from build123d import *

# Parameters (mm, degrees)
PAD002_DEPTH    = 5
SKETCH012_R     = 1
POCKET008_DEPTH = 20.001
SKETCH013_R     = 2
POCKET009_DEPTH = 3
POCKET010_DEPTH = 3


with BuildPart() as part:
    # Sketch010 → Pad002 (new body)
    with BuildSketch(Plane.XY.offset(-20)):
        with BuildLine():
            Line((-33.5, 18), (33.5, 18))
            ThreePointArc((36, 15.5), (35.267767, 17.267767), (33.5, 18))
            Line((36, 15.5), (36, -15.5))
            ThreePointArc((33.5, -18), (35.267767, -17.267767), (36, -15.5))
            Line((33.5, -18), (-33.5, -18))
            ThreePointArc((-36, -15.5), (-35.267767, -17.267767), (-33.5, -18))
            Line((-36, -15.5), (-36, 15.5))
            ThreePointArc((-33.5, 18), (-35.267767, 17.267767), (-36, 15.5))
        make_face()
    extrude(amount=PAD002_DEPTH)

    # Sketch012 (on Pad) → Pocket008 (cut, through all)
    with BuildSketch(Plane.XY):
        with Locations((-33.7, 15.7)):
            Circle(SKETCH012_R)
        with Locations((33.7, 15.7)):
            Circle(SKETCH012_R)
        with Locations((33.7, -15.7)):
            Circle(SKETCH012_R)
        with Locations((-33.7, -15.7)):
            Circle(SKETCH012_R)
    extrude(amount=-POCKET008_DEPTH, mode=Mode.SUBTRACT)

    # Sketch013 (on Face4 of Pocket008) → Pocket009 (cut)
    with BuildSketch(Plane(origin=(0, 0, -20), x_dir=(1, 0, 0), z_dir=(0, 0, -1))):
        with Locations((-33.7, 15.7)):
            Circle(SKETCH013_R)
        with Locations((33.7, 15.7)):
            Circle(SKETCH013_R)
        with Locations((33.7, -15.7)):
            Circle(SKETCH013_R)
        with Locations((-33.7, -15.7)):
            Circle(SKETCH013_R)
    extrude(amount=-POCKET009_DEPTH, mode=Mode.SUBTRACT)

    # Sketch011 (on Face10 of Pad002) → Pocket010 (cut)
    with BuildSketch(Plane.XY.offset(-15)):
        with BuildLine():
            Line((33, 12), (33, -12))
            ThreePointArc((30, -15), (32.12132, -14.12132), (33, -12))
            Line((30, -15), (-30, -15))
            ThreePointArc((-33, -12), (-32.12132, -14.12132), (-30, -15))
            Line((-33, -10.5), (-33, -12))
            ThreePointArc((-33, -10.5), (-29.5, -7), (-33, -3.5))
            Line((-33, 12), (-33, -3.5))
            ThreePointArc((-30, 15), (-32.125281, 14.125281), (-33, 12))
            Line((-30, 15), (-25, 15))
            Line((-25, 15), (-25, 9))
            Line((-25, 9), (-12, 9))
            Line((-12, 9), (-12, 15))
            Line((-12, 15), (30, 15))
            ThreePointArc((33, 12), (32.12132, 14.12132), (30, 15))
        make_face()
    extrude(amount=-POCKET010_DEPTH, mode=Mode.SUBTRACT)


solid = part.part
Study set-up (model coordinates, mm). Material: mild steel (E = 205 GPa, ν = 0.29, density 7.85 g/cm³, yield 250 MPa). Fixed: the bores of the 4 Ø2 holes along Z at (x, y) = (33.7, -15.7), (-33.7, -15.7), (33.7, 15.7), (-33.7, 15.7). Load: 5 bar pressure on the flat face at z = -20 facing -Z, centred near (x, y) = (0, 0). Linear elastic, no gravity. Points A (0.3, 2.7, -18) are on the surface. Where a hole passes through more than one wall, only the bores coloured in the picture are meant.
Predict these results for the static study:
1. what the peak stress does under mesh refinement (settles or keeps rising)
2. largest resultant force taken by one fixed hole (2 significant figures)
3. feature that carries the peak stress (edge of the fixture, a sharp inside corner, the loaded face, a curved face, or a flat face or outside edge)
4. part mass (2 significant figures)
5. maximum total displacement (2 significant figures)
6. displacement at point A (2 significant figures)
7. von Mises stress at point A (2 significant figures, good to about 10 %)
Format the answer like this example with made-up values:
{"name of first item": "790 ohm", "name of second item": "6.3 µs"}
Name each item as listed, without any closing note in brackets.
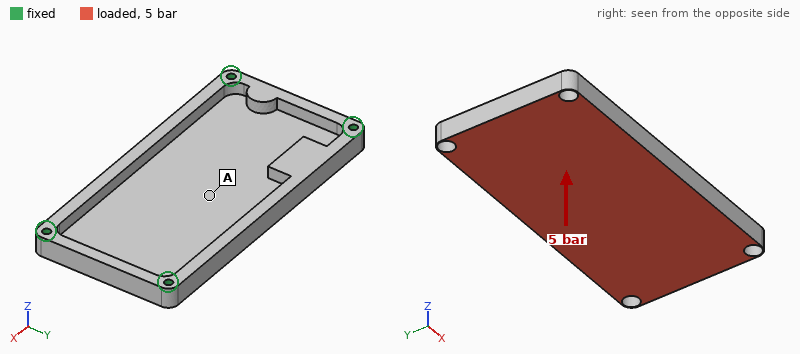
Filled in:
{"what the peak stress does under mesh refinement": "keeps rising", "largest resultant force taken by one fixed hole": "790 N", "feature that carries the peak stress": "edge of the fixture", "part mass": "56 g", "maximum total displacement": "78 µm", "displacement at point A": "77 µm", "von Mises stress at point A": "41 MPa"}
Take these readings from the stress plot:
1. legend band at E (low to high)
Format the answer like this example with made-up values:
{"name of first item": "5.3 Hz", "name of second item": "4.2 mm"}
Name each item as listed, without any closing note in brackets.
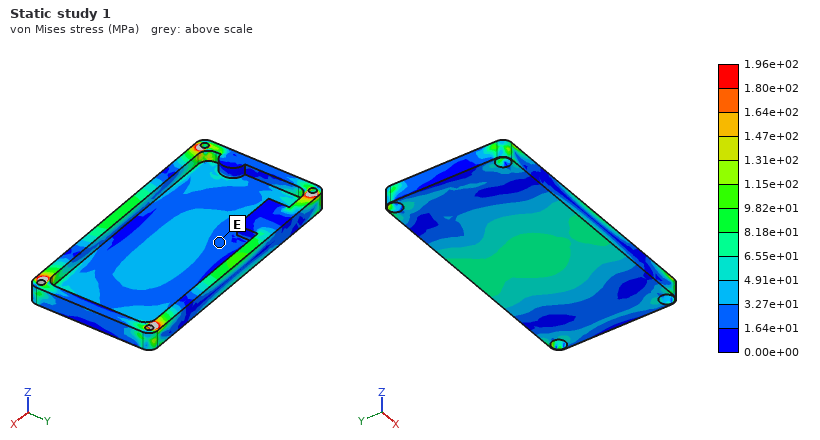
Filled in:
{"legend band at E": "1.64e+01 to 3.27e+01 MPa"}
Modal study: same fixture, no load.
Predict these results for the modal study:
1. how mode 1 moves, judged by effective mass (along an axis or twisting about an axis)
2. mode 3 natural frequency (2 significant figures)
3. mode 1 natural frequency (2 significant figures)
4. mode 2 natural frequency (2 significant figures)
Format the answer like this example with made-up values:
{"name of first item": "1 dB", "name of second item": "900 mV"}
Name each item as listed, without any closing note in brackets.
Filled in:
{"how mode 1 moves, judged by effective mass": "along Z", "mode 3 natural frequency": "7900 Hz", "mode 1 natural frequency": "3500 Hz", "mode 2 natural frequency": "5000 Hz"}
